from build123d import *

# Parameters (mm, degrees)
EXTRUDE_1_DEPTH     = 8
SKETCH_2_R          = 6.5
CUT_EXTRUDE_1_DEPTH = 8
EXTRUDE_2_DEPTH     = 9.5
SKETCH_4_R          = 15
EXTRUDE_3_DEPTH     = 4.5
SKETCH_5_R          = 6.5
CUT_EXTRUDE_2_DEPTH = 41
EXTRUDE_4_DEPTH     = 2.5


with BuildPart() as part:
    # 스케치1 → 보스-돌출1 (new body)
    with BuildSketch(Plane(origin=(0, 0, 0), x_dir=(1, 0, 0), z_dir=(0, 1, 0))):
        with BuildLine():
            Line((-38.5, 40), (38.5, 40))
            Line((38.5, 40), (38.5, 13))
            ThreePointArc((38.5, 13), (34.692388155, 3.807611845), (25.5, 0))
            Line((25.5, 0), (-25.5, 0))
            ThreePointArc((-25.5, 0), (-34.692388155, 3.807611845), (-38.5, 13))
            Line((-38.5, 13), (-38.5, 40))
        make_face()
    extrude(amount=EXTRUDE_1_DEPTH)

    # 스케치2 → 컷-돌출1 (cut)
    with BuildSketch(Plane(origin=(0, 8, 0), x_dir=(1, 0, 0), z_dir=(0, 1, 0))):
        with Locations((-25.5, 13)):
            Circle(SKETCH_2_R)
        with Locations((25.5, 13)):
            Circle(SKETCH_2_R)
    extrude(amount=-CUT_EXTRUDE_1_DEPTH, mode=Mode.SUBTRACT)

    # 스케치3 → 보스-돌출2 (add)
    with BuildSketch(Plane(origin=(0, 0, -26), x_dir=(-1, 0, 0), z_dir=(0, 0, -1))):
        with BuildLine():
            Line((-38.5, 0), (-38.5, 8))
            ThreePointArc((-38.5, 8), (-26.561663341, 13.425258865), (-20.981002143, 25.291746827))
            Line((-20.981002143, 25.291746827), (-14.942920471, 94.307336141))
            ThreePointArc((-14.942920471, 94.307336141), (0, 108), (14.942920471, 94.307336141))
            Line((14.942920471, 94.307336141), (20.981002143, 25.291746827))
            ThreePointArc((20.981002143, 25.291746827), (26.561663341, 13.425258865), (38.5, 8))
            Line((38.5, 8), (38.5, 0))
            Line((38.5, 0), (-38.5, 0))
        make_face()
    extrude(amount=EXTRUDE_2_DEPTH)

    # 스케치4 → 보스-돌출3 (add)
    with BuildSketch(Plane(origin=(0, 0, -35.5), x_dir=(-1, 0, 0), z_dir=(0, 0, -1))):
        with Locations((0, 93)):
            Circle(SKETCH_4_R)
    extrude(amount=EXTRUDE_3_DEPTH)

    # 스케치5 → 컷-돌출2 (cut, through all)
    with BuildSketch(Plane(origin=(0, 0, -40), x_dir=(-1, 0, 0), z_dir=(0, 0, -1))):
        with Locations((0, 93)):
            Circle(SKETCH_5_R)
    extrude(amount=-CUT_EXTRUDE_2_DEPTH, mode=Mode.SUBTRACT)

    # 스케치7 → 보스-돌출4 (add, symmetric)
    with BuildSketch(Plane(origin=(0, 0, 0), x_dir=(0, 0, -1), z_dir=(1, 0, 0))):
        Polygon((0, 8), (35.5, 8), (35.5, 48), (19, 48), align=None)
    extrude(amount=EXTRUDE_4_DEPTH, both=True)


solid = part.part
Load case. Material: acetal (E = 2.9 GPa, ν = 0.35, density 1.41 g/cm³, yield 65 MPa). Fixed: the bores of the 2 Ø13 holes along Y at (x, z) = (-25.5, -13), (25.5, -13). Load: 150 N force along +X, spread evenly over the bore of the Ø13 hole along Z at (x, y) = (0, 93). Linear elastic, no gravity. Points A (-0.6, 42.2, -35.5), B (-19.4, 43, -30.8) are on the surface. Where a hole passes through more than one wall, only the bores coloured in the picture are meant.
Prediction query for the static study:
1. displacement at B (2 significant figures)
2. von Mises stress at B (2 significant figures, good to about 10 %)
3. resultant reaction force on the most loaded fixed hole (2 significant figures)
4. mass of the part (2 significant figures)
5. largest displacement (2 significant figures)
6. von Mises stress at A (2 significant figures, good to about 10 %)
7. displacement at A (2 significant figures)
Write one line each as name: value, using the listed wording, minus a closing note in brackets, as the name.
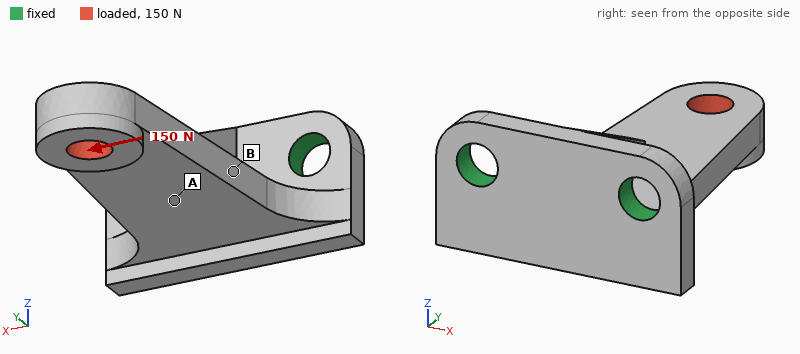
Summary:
displacement at B: 0.13 mm
von Mises stress at B: 3.2 MPa
resultant reaction force on the most loaded fixed hole: 280 N
mass of the part: 87 g
largest displacement: 0.47 mm
von Mises stress at A: 1.3 MPa
displacement at A: 0.10 mm
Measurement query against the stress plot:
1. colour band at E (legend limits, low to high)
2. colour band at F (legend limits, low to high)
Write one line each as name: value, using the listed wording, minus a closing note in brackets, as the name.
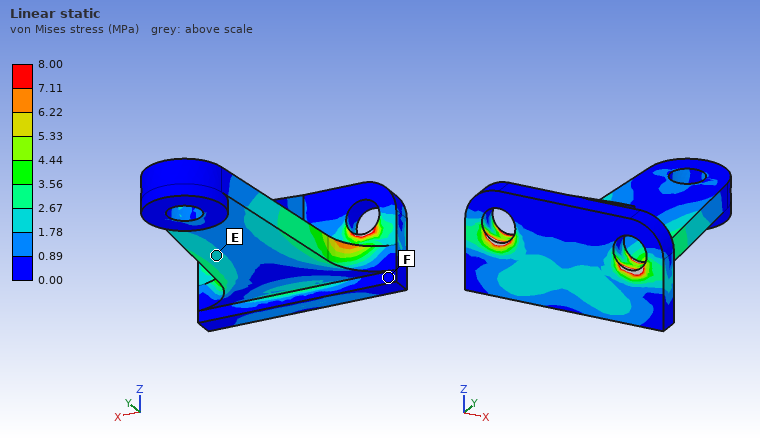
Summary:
colour band at E: 1.78 to 2.67 MPa
colour band at F: 0.00 to 0.89 MPa
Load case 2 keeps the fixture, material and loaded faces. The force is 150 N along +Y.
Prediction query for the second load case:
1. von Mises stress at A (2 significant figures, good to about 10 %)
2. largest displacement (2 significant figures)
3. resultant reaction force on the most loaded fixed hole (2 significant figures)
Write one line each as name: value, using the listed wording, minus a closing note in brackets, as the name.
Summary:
von Mises stress at A: 0.83 MPa
largest displacement: 0.28 mm
resultant reaction force on the most loaded fixed hole: 77 N
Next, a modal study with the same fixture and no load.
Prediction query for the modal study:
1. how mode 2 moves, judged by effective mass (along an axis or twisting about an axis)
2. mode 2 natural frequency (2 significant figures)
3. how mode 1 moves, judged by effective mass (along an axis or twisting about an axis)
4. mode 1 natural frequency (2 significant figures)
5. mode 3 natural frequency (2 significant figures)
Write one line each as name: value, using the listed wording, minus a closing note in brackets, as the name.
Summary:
how mode 2 moves, judged by effective mass: along X
mode 2 natural frequency: 730 Hz
how mode 1 moves, judged by effective mass: along Z
mode 1 natural frequency: 310 Hz
mode 3 natural frequency: 1200 Hz
